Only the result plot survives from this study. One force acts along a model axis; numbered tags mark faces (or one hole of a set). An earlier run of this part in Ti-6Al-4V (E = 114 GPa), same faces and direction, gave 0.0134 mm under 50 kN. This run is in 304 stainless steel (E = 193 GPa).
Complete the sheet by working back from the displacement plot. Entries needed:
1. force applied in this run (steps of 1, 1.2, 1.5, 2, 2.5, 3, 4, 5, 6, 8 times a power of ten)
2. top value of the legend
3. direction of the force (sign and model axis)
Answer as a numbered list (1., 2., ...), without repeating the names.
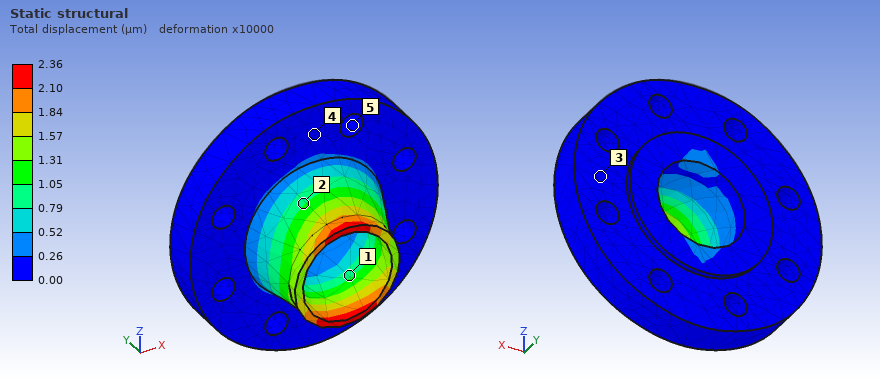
1. 15 kN
2. 2.36 µm
3. -Z
